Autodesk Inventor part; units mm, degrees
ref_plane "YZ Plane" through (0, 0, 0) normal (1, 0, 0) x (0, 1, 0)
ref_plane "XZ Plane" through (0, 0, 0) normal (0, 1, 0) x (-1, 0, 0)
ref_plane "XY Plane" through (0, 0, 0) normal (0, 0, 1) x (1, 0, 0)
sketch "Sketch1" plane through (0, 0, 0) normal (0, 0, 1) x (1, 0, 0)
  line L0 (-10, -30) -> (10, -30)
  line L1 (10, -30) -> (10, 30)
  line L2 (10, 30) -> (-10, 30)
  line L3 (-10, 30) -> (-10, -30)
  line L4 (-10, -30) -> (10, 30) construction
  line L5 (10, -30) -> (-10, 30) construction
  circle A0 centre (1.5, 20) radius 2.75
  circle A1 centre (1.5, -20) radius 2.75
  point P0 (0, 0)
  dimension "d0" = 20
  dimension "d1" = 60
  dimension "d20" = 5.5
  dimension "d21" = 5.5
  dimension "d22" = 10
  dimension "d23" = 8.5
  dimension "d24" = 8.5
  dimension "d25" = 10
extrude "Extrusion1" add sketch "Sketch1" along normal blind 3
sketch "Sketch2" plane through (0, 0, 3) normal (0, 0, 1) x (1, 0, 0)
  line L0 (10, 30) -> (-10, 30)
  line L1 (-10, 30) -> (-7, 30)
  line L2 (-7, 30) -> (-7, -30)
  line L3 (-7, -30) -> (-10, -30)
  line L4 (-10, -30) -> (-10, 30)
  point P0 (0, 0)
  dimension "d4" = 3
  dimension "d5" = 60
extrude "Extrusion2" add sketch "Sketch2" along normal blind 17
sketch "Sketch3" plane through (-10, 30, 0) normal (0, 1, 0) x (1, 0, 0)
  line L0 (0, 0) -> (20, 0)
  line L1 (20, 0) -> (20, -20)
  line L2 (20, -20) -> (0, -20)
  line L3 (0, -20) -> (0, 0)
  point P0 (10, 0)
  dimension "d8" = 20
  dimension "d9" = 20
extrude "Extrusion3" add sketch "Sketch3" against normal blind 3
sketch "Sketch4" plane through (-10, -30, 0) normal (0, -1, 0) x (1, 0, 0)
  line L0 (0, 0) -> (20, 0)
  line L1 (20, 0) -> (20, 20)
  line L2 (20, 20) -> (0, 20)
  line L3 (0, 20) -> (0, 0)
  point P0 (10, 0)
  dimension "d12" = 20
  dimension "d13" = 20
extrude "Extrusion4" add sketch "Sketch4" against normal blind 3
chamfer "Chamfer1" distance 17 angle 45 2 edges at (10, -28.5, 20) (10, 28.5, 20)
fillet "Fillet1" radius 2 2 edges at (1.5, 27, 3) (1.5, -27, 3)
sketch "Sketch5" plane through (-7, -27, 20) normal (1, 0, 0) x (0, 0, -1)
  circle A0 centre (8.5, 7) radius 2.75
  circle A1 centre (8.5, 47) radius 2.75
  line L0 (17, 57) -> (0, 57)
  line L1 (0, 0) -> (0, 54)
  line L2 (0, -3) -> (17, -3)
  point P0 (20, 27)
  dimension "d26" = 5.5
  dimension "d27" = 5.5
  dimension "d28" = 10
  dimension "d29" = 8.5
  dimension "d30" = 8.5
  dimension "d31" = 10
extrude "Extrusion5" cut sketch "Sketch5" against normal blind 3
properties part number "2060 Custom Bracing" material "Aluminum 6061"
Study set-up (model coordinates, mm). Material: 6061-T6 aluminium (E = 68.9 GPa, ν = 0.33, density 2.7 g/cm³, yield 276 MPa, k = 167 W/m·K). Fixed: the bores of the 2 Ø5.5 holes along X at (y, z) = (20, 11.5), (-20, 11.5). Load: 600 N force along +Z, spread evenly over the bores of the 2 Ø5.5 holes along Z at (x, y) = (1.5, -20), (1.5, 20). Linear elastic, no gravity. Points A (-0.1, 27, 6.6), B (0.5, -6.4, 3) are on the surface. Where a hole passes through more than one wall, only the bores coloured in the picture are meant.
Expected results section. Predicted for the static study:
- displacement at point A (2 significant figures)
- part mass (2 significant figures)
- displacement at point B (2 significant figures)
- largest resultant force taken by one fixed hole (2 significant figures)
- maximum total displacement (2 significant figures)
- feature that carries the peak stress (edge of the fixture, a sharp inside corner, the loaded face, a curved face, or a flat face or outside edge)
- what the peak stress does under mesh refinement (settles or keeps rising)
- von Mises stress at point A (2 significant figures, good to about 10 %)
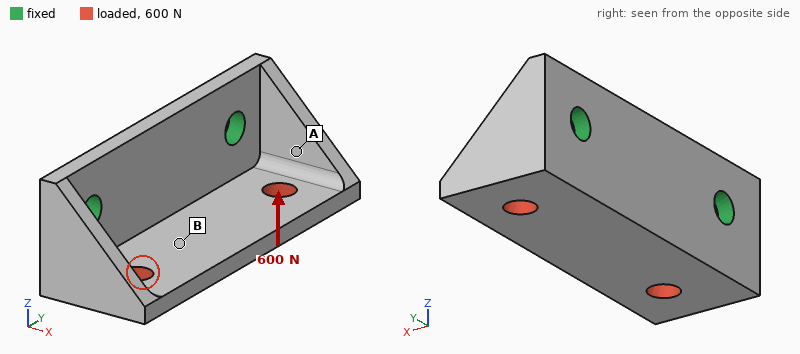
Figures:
24 µm
20 g
35 µm
310 N
75 µm
edge of the fixture
keeps rising
25 MPa
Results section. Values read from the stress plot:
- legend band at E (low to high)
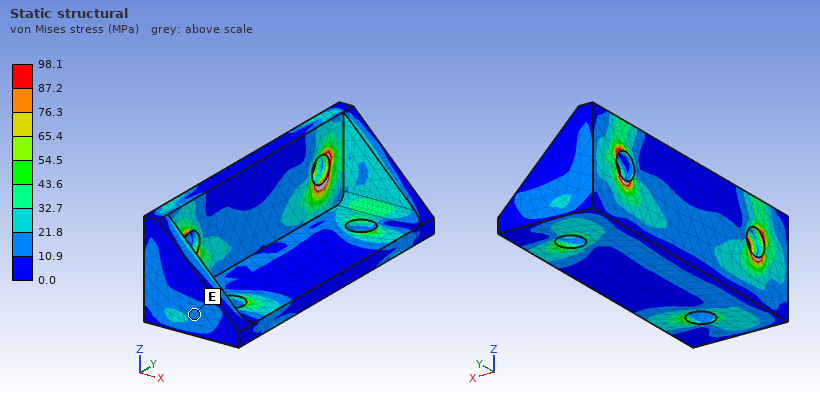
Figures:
10.9 to 21.8 MPa
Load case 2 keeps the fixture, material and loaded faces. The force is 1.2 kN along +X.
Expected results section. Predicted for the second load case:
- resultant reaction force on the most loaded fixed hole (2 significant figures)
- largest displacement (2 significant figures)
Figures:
600 N
81 µm
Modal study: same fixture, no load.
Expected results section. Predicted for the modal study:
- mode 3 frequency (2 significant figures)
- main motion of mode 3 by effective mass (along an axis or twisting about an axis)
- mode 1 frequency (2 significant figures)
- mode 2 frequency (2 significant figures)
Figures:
10 kHz
along X
5200 Hz
7200 Hz
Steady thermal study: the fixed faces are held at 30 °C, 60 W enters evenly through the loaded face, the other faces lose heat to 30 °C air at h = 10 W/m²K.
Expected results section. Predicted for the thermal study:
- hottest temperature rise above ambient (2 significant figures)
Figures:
46 K
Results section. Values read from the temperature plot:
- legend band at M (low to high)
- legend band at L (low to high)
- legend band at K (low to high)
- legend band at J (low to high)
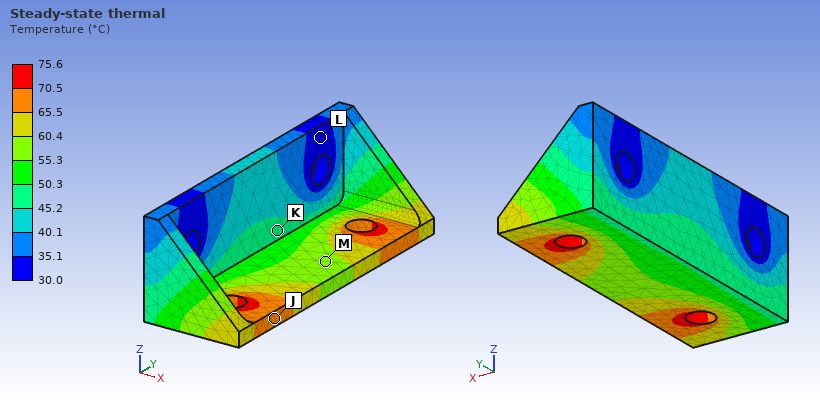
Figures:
55.3 to 60.4 °C
30.0 to 35.1 °C
45.2 to 50.3 °C
65.5 to 70.5 °C
